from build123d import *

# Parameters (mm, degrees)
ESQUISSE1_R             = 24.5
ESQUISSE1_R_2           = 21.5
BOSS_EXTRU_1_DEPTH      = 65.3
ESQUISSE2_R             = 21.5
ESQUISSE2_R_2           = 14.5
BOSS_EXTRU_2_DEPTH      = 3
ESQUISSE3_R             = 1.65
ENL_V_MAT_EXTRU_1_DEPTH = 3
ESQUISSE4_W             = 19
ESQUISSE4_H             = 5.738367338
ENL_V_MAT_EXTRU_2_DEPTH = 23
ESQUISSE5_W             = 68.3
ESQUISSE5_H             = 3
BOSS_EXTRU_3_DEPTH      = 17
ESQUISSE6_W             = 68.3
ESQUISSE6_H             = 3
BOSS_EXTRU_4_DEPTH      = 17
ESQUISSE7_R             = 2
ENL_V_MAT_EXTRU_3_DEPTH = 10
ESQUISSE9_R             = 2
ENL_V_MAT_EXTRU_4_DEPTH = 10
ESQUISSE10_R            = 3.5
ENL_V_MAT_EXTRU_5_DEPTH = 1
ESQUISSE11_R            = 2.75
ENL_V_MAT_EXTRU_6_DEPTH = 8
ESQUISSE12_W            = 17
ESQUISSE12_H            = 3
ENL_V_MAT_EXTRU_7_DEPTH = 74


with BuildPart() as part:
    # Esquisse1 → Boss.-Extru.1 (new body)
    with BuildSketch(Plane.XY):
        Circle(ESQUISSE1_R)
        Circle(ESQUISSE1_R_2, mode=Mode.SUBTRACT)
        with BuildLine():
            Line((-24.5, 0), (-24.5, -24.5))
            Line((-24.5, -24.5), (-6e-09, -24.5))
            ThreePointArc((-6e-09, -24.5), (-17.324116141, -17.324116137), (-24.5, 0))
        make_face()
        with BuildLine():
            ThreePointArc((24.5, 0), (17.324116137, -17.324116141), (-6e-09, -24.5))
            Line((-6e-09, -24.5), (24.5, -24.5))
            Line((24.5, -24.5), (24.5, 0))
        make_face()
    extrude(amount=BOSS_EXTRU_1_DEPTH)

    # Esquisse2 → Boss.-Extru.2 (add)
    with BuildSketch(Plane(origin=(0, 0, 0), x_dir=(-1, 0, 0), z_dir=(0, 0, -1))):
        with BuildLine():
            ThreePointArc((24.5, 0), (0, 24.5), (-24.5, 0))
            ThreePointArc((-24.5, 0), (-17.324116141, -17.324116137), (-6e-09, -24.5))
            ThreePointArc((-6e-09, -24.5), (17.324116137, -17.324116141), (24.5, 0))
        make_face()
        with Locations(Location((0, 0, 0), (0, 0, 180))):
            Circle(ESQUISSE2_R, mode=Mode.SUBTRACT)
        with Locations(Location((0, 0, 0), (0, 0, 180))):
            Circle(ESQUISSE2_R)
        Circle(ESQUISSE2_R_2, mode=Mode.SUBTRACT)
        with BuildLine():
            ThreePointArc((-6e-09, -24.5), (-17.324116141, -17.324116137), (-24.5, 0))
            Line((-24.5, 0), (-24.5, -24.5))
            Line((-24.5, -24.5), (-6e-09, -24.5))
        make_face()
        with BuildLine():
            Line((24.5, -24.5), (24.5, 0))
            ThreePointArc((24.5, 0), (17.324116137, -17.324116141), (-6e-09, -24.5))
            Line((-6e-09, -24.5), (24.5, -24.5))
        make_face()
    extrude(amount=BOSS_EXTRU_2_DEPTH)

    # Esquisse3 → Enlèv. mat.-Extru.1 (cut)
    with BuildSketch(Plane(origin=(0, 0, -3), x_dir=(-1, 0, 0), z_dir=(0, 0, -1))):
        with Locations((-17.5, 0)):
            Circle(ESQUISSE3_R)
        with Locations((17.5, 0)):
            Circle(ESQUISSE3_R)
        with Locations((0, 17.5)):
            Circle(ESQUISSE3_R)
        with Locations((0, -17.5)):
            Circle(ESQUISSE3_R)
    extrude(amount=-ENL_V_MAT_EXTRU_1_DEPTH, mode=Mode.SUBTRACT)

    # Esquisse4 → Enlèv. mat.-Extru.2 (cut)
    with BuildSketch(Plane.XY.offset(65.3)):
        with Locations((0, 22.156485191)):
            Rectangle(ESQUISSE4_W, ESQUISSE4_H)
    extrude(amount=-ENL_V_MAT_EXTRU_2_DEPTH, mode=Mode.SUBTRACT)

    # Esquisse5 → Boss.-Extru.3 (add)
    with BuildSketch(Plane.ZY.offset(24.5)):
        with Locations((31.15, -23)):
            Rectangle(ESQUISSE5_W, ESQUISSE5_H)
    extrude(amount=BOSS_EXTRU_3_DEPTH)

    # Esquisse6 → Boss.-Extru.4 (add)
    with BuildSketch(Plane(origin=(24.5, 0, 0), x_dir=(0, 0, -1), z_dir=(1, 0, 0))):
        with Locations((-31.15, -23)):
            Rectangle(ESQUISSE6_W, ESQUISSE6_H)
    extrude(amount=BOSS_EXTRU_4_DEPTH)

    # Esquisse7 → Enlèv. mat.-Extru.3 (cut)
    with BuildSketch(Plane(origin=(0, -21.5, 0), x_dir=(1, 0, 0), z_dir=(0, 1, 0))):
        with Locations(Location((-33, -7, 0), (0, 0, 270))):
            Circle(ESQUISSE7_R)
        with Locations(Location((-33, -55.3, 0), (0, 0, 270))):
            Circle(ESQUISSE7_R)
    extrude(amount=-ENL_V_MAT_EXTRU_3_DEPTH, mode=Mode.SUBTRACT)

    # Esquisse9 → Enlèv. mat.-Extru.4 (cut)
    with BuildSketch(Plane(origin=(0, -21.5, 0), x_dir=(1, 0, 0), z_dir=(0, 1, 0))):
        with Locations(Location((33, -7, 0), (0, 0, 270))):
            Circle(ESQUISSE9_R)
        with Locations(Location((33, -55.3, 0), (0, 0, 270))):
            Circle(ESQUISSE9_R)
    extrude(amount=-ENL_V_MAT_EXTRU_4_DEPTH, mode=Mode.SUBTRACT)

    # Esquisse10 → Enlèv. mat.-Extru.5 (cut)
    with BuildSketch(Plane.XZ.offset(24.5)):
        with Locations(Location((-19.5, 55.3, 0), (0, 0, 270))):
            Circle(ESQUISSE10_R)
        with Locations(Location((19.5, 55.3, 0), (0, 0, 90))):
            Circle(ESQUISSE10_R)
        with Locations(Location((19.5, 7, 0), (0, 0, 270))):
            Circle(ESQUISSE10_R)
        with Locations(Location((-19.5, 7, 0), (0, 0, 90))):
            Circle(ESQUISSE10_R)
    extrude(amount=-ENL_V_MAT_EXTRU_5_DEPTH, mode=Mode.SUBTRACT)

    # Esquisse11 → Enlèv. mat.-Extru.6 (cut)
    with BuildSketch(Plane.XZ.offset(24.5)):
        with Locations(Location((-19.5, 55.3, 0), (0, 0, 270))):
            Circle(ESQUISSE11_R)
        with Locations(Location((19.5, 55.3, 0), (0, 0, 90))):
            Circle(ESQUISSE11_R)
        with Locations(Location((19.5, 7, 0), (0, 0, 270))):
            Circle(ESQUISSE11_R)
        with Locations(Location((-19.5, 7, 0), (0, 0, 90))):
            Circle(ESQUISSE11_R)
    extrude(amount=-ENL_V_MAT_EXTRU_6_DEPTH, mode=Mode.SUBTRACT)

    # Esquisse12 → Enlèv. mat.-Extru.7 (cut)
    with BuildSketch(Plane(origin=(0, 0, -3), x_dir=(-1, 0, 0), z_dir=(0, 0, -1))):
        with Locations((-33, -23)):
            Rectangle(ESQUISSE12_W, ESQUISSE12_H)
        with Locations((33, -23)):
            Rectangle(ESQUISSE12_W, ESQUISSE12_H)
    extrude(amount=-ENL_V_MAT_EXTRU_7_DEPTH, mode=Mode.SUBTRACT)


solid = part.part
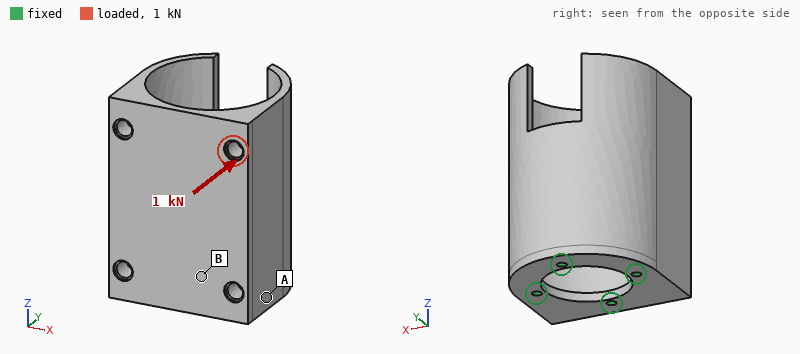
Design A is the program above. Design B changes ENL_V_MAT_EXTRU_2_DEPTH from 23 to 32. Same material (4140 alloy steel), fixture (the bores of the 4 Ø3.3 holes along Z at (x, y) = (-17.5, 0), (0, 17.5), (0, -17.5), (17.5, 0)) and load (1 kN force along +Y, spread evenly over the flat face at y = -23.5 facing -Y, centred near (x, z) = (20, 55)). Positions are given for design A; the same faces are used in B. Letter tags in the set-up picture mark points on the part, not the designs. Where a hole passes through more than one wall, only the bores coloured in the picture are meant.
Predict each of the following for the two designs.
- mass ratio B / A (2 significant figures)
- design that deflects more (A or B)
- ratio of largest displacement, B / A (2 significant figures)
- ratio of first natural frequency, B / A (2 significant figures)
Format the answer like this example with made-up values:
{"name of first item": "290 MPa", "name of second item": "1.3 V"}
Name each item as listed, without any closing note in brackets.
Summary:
{"mass ratio B / A": "0.99", "design that deflects more": "B", "ratio of largest displacement, B / A": "1.2", "ratio of first natural frequency, B / A": "0.98"}
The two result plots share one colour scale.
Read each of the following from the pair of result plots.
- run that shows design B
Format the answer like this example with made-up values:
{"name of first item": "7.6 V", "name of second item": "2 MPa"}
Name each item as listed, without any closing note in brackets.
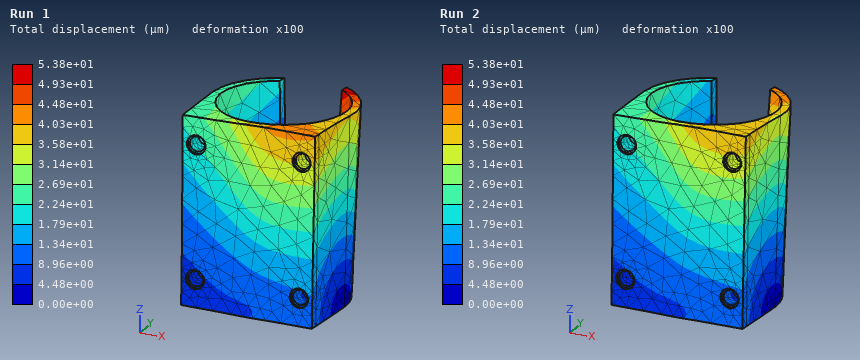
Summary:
{"run that shows design B": "Run 1"}
